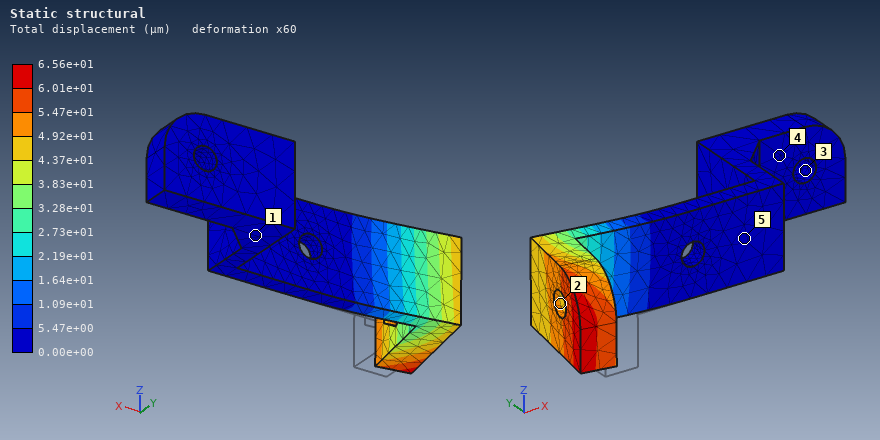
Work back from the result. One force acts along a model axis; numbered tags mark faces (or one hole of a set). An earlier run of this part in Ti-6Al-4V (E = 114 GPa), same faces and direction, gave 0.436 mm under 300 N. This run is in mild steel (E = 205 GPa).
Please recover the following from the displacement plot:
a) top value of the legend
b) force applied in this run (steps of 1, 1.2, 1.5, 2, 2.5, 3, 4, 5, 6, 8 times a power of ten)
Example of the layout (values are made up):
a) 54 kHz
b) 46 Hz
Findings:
a) 6.56e+01 µm
b) 80 N
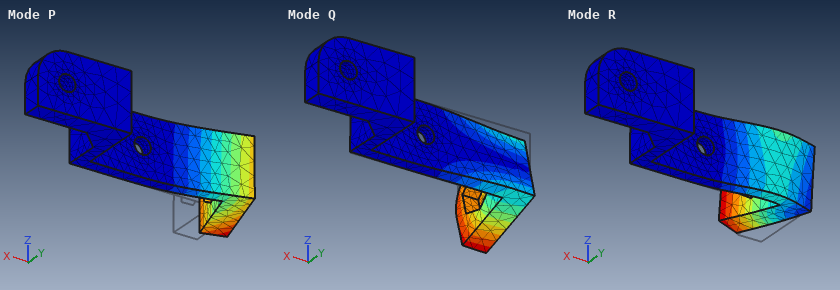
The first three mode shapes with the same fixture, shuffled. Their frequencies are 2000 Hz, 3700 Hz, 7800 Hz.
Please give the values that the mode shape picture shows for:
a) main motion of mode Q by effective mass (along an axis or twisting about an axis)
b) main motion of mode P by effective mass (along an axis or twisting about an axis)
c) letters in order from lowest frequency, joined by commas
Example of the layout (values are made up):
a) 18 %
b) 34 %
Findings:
a) along Z
b) along Y
c) P, Q, R
